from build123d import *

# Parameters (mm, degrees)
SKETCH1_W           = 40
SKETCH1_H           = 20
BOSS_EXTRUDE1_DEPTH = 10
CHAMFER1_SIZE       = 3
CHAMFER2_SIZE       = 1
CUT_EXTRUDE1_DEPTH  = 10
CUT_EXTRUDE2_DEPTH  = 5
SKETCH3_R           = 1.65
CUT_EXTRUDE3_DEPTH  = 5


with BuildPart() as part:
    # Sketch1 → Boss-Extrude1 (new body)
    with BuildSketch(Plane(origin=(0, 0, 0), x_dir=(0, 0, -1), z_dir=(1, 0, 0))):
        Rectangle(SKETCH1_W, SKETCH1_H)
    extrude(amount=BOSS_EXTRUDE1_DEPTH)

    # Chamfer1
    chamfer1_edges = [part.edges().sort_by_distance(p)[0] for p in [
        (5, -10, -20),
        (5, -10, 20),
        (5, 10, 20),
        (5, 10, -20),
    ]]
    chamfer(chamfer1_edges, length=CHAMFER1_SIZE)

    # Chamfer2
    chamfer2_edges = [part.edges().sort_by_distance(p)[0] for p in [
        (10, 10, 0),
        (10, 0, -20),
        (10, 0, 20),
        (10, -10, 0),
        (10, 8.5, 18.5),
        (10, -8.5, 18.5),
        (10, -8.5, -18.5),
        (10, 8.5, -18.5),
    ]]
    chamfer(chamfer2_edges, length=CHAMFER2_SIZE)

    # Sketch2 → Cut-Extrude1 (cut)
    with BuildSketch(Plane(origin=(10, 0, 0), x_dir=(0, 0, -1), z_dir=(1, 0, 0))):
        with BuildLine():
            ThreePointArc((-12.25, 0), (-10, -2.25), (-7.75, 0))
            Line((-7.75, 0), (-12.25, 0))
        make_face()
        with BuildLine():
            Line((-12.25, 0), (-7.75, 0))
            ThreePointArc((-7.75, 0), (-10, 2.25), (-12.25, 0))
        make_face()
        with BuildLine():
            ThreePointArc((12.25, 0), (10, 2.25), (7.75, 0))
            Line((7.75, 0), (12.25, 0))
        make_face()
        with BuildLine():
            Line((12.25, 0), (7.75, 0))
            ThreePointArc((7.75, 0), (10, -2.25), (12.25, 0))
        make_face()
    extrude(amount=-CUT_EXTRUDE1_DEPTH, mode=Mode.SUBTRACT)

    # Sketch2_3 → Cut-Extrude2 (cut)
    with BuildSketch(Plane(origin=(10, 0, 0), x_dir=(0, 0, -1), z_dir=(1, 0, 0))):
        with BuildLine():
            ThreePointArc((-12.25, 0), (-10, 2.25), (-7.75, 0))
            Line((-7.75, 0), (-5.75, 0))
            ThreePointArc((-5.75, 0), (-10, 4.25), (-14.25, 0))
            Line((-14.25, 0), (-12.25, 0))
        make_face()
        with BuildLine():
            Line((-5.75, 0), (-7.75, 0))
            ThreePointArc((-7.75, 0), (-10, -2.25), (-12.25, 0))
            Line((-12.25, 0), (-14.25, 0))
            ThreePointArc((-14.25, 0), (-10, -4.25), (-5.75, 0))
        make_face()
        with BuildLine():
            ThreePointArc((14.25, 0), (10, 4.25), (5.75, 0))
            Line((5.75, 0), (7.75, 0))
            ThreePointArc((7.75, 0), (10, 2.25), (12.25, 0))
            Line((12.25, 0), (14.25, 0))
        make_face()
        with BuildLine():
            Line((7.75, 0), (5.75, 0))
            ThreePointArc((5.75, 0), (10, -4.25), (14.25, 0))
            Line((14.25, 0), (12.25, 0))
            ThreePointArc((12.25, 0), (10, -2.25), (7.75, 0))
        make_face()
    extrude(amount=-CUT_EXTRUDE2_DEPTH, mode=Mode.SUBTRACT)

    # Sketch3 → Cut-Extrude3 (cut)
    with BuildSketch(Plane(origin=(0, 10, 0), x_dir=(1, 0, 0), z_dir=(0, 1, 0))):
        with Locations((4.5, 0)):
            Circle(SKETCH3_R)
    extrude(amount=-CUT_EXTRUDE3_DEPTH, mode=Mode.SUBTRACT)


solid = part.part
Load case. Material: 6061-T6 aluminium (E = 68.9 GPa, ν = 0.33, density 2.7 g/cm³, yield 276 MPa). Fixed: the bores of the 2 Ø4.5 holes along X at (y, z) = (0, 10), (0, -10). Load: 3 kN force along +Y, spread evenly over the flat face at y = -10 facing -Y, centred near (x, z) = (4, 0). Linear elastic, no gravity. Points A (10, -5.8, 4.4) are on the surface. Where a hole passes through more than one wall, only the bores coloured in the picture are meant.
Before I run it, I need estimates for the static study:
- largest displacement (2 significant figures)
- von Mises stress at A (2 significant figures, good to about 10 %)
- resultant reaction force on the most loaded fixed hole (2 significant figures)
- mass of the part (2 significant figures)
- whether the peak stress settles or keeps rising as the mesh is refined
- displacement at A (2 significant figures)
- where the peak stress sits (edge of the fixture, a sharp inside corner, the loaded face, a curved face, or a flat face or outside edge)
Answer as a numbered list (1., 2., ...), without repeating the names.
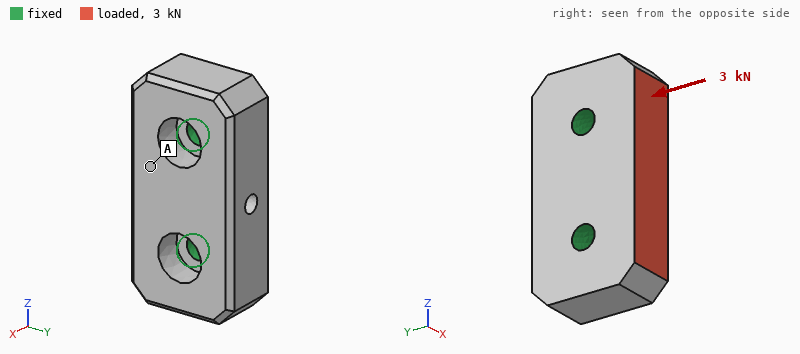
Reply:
1. 7.3 µm
2. 8.2 MPa
3. 1.5 kN
4. 19 g
5. keeps rising
6. 6.3 µm
7. edge of the fixture
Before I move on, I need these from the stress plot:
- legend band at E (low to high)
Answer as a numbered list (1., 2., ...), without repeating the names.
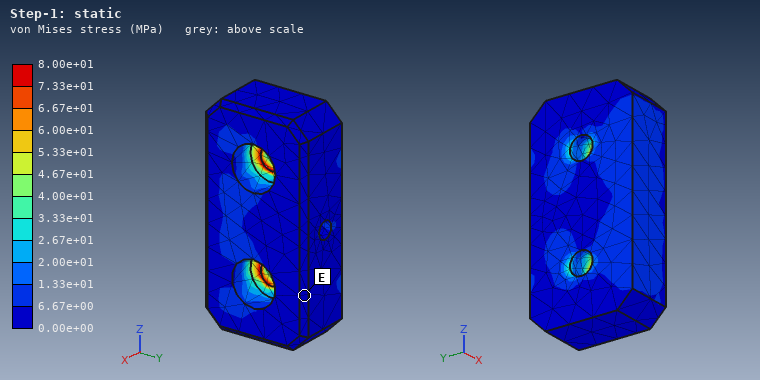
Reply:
1. 0.00e+00 to 6.67e+00 MPa
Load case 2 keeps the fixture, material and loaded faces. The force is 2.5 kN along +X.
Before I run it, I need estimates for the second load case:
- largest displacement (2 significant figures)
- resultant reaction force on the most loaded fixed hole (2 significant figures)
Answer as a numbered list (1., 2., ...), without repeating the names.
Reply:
1. 27 µm
2. 1.3 kN
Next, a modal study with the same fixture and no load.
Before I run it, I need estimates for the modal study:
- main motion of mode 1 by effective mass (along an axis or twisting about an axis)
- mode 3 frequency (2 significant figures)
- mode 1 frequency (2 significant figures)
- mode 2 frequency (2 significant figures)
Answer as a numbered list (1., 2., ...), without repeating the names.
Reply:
1. along Y
2. 31 kHz
3. 20 kHz
4. 30 kHz
